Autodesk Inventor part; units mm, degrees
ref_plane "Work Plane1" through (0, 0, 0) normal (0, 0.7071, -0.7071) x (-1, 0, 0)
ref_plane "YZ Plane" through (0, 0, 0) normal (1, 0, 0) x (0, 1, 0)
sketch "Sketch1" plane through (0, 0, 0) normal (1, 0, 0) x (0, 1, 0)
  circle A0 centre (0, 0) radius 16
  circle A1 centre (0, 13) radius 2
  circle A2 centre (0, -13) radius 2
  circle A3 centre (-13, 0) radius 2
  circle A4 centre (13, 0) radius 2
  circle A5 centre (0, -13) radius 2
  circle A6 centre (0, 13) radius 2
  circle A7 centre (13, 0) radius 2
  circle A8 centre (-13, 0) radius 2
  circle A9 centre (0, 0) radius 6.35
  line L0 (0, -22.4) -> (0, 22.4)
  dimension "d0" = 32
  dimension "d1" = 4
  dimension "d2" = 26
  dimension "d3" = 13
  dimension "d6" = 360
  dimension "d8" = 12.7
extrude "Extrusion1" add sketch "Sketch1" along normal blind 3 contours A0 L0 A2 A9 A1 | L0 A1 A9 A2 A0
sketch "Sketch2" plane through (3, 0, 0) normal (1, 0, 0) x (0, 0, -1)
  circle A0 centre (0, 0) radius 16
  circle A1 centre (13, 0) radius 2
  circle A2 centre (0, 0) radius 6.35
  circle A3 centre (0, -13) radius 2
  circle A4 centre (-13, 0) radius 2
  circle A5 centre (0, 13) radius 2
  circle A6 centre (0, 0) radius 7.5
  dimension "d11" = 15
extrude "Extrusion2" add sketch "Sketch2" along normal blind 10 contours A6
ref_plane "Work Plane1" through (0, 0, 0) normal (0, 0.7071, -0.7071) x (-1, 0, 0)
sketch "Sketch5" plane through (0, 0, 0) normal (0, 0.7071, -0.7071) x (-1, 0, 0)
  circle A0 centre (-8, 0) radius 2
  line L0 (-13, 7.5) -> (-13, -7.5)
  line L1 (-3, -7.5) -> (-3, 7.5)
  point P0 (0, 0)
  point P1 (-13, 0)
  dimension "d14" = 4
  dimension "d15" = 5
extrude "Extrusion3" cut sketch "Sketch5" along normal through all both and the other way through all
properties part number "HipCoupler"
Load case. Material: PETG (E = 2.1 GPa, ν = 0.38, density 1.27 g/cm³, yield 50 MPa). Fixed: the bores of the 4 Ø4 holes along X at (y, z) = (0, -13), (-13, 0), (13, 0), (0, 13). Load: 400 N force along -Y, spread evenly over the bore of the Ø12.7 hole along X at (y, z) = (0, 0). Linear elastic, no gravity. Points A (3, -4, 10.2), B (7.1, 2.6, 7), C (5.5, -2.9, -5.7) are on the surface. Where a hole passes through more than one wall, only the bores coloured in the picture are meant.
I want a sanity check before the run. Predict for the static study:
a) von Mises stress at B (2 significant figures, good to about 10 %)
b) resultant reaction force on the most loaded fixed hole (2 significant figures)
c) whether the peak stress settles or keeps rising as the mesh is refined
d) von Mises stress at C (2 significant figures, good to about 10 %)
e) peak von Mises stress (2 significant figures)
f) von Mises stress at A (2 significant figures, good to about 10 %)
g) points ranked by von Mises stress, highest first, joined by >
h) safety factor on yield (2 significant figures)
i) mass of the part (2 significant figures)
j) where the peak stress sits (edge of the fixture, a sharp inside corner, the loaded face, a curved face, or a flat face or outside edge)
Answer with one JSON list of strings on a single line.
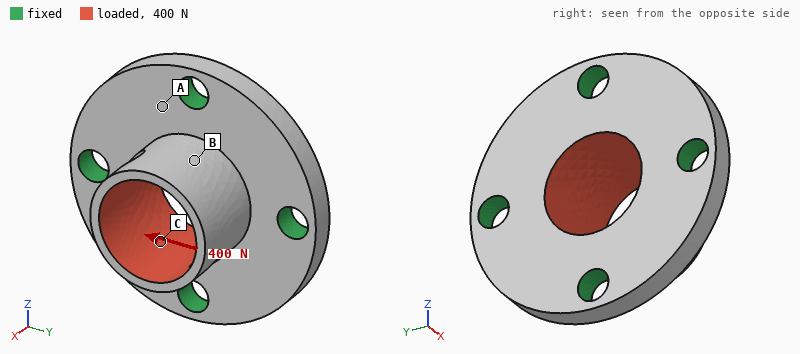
["11 MPa", "150 N", "settles", "17 MPa", "36 MPa", "3.2 MPa", "C > B > A", "1.4", "3.0 g", "the loaded face"]
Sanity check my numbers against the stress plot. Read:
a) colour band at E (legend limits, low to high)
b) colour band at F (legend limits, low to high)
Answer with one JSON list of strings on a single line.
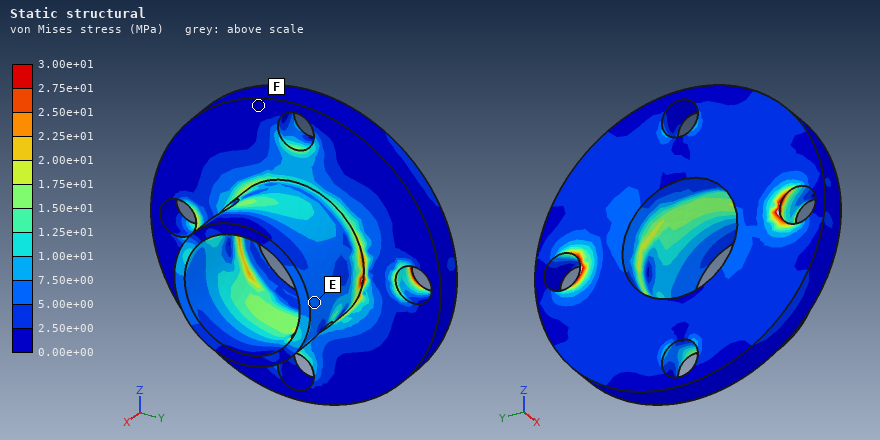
["5.00e+00 to 7.50e+00 MPa", "0.00e+00 to 2.50e+00 MPa"]
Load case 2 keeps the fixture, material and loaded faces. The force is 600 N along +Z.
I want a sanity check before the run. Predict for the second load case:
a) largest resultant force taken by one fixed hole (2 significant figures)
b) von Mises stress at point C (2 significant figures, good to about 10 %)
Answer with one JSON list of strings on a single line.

["220 N", "16 MPa"]
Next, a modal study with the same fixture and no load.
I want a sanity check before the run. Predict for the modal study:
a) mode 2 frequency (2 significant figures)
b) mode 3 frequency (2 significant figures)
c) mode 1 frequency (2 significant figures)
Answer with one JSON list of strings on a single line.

["7000 Hz", "7700 Hz", "6700 Hz"]
